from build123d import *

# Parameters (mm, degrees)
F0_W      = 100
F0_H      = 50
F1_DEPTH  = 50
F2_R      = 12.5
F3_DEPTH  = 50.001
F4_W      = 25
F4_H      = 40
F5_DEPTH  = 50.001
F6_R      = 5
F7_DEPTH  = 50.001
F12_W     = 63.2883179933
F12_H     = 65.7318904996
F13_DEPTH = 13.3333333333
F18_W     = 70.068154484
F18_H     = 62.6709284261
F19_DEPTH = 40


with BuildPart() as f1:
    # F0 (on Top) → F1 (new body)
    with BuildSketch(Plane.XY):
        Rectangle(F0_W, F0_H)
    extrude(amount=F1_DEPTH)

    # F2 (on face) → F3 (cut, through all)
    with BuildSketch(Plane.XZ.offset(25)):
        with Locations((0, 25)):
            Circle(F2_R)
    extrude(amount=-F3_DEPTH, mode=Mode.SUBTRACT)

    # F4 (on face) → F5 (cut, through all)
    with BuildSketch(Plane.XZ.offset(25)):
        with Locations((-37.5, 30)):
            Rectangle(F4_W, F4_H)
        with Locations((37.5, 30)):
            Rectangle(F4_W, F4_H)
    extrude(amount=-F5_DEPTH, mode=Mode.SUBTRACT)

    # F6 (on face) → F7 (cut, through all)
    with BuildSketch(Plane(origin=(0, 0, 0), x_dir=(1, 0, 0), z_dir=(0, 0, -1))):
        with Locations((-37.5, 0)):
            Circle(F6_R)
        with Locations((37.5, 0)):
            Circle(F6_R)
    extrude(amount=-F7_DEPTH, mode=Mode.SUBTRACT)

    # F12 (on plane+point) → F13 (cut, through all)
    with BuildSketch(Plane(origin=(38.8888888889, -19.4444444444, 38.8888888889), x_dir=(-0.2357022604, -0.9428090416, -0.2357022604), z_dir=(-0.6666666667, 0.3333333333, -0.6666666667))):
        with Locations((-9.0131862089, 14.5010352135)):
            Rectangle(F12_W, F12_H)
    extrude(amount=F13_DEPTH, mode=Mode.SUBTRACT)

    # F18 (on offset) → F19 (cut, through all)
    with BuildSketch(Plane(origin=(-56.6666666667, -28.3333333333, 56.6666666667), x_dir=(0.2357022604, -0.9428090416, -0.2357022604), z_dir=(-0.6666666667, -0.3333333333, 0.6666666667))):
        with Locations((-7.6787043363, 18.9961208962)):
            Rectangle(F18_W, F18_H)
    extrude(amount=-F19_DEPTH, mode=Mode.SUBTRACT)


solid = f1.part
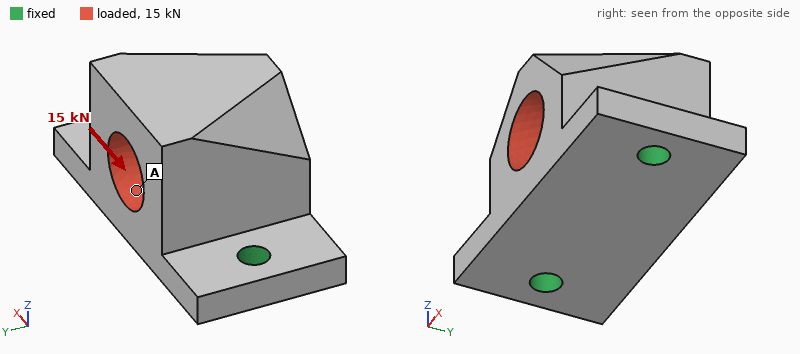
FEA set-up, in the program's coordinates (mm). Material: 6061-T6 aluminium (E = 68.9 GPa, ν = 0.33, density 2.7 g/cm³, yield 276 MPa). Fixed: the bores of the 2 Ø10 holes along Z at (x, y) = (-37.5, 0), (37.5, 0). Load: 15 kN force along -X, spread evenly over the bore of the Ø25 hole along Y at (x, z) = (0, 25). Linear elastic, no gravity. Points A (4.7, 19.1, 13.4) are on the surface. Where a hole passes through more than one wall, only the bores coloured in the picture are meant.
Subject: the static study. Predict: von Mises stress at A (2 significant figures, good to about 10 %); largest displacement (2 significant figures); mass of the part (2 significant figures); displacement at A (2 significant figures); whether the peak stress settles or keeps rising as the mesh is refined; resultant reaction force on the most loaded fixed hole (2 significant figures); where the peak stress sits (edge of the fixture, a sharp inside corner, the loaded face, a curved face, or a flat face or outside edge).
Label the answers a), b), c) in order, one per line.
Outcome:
a) 16 MPa
b) 46 µm
c) 320 g
d) 11 µm
e) keeps rising
f) 8.9 kN
g) edge of the fixture
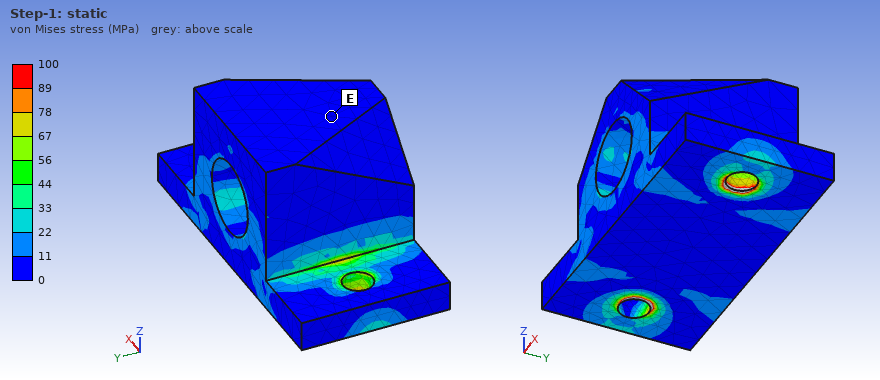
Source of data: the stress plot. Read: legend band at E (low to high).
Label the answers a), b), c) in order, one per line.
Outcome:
a) 0 to 11 MPa
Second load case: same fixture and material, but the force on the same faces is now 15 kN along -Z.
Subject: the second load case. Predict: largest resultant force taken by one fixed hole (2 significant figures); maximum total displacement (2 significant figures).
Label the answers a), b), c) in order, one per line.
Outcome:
a) 8.0 kN
b) 40 µm
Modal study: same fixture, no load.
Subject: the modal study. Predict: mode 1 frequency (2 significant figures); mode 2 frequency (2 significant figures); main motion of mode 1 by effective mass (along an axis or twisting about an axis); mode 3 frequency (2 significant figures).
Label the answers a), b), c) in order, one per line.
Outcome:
a) 2600 Hz
b) 6400 Hz
c) along Y
d) 6700 Hz
